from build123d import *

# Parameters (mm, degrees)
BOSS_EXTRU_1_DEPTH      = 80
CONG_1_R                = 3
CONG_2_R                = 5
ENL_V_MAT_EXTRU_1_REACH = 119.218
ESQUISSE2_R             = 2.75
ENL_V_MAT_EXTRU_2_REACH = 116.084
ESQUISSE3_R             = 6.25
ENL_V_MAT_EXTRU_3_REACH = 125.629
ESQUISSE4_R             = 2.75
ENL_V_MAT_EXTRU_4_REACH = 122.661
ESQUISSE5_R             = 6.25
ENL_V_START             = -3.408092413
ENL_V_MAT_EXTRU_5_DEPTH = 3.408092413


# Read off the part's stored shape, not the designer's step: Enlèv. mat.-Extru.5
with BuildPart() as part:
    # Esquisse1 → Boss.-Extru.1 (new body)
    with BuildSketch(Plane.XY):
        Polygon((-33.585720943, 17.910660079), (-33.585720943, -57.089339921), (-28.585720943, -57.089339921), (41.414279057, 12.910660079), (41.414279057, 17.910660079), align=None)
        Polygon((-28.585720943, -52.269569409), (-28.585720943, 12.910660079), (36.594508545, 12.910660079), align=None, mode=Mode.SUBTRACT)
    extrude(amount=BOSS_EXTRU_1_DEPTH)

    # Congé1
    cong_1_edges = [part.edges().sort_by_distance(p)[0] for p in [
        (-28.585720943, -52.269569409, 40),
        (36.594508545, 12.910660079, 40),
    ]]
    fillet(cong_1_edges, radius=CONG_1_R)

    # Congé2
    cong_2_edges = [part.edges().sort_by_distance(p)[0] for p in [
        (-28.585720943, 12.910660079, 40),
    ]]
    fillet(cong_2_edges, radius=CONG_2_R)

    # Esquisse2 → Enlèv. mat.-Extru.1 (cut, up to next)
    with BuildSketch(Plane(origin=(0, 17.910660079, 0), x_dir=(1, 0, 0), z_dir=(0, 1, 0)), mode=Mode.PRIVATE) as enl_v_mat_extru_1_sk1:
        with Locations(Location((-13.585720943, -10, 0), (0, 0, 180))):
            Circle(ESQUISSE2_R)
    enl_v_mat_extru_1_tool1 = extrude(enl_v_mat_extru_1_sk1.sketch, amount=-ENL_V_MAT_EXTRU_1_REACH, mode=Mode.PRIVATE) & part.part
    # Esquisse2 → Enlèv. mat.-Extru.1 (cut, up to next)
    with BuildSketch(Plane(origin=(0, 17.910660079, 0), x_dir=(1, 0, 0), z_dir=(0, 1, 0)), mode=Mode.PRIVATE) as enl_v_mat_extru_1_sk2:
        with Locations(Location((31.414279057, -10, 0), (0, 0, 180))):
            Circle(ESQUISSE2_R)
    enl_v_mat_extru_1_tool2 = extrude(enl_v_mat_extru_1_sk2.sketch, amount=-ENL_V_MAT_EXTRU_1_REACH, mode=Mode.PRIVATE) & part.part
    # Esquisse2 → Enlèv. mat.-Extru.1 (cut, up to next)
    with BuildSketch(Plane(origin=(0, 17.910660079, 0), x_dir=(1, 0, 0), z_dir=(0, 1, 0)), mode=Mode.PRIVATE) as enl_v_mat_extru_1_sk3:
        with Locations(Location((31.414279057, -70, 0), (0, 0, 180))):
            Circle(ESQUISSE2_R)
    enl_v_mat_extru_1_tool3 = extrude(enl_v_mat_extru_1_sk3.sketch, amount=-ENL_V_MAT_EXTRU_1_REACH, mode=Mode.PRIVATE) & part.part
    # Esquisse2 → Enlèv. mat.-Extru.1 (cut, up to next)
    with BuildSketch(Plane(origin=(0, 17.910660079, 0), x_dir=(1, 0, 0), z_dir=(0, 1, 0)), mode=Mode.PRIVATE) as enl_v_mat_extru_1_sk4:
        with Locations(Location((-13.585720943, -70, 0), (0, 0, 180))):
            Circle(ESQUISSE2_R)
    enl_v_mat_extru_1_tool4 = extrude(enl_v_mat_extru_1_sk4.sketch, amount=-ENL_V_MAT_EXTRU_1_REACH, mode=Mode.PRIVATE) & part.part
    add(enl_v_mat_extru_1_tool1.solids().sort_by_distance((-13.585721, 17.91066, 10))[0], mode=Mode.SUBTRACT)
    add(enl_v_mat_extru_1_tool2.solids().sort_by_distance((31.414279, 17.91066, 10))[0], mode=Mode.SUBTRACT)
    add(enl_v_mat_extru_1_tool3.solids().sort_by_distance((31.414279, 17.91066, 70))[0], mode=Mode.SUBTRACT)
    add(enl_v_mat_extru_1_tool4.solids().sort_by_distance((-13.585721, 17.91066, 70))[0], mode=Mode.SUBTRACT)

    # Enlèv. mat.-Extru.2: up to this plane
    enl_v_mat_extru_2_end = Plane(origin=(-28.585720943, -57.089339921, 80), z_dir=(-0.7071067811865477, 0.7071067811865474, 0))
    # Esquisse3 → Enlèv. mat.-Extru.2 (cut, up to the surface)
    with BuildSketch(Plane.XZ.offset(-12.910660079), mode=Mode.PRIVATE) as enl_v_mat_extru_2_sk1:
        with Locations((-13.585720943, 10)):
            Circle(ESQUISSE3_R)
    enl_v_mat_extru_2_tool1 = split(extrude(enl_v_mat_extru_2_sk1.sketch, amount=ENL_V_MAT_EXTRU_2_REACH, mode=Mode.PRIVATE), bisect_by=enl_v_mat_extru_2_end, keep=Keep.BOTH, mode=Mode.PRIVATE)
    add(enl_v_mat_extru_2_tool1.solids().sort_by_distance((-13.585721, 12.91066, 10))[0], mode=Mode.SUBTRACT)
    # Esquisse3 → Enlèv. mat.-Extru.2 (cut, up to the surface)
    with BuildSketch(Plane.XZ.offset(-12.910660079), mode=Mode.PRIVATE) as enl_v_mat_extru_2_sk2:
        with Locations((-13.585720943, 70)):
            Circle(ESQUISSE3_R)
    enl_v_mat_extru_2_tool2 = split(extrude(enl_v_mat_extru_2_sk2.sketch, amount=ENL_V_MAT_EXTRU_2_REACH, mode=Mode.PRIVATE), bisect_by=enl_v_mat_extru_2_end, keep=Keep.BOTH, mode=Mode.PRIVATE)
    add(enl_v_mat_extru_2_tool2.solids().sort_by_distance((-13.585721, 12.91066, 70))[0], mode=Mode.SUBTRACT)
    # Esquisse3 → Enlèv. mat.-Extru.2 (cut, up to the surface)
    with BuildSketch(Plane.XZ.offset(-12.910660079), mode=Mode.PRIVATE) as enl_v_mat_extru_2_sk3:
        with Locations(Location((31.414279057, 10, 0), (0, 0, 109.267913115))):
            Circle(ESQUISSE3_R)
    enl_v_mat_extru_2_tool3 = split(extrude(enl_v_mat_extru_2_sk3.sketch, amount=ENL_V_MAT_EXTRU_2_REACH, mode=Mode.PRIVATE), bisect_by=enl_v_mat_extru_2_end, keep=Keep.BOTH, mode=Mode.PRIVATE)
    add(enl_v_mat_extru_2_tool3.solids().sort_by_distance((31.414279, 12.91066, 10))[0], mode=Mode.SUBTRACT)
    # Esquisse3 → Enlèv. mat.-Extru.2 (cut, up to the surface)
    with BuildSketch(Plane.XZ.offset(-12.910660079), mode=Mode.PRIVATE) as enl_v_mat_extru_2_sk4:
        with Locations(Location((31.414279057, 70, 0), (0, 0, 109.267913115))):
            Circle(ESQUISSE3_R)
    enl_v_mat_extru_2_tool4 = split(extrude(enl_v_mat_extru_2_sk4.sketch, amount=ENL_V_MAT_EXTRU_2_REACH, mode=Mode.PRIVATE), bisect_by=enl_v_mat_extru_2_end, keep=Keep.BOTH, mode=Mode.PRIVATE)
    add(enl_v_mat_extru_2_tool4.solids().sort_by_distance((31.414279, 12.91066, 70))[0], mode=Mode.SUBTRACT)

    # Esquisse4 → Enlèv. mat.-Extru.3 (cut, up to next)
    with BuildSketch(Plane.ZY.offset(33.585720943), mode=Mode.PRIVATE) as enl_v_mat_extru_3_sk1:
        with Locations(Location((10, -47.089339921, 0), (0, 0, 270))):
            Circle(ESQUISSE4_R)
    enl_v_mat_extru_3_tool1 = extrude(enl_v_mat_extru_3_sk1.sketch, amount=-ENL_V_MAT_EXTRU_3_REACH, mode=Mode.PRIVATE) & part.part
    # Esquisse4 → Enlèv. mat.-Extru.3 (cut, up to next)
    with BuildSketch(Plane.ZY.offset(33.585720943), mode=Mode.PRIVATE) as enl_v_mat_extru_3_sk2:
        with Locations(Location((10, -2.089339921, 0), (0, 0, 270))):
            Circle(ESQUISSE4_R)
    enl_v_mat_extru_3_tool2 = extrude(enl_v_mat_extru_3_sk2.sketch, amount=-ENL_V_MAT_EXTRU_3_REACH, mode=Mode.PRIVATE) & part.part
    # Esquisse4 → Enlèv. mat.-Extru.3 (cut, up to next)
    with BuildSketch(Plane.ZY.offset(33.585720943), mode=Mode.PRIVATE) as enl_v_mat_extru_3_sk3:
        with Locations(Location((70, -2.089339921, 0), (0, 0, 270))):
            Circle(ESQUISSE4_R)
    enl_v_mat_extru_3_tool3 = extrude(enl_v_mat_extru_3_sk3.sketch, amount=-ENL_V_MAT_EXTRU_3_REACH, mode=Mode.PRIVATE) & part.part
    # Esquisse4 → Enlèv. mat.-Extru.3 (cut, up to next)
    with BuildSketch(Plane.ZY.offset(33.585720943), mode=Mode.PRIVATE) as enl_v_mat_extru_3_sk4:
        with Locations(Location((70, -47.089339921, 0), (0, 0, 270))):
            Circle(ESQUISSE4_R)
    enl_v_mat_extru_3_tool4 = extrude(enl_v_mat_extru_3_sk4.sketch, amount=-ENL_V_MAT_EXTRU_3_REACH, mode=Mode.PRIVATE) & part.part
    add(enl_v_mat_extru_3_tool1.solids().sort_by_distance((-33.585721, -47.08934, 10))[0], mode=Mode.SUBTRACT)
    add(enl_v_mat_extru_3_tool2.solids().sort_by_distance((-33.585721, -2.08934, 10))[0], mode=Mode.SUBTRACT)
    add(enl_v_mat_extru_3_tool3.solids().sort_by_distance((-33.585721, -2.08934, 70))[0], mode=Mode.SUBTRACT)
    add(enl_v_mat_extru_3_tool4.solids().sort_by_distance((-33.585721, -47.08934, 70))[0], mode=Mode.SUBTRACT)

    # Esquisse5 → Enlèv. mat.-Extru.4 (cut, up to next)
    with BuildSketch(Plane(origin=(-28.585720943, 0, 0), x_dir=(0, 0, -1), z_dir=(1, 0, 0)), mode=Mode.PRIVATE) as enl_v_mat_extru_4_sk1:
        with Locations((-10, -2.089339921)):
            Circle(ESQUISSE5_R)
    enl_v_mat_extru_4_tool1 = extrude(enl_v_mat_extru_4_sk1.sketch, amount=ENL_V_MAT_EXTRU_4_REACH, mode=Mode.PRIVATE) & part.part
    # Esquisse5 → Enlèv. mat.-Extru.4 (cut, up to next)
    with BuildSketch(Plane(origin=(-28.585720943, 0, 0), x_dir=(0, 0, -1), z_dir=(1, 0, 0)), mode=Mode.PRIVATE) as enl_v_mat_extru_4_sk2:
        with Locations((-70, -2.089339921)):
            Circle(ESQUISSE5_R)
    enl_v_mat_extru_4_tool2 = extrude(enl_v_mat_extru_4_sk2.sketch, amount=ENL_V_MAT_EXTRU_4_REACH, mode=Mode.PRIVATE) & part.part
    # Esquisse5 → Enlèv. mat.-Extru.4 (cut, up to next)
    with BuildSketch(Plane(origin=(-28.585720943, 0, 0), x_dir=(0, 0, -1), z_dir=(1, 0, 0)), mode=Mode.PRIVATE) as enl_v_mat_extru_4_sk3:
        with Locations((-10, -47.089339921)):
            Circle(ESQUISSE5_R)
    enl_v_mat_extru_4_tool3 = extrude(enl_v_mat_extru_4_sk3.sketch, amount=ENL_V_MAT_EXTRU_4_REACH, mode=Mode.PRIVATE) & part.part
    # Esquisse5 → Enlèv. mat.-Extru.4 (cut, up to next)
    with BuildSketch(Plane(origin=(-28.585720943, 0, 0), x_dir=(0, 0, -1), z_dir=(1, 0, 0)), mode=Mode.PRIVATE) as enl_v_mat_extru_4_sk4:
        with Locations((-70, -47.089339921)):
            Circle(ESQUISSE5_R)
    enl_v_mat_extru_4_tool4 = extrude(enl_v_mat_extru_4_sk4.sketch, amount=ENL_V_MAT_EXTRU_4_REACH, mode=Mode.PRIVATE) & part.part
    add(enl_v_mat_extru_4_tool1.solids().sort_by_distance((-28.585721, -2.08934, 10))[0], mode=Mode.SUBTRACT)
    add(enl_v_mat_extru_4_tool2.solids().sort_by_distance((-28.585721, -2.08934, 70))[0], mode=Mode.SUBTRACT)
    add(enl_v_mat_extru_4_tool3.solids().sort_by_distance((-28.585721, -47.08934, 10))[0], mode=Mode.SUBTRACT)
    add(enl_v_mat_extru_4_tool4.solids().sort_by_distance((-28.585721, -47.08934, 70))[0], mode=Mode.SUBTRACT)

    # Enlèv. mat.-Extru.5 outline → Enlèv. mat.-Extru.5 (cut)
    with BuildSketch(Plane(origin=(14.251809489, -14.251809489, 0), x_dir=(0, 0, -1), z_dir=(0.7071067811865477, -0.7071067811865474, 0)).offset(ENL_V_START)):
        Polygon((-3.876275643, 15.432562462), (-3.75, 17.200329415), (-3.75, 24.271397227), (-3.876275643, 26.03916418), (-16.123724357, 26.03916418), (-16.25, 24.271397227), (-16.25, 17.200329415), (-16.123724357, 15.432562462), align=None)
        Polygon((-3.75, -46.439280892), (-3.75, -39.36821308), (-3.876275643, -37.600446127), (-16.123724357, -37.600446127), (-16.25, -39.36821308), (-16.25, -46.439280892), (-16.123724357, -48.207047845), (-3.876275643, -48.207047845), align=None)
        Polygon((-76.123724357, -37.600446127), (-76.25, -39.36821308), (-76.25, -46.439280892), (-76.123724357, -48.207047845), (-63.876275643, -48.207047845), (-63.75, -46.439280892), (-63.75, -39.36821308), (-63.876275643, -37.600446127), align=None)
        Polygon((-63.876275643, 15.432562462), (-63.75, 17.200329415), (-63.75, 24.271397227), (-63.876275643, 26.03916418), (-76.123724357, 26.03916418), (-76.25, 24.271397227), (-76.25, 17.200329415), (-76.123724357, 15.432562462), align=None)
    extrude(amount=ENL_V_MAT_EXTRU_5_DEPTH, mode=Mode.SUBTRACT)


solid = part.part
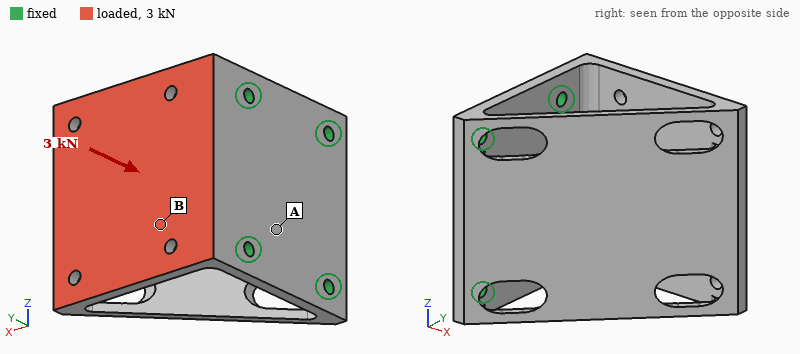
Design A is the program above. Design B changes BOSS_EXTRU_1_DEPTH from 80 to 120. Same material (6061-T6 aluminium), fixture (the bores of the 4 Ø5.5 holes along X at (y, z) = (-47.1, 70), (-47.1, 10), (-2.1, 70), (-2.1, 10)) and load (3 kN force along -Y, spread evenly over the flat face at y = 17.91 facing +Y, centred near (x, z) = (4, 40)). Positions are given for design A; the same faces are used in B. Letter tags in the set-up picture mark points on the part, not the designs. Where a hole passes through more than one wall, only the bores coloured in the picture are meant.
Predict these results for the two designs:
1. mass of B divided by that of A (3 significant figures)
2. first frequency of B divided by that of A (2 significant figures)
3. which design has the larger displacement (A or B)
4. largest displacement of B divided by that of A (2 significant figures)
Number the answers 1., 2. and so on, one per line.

1. 1.53
2. 0.94
3. A
4. 0.72
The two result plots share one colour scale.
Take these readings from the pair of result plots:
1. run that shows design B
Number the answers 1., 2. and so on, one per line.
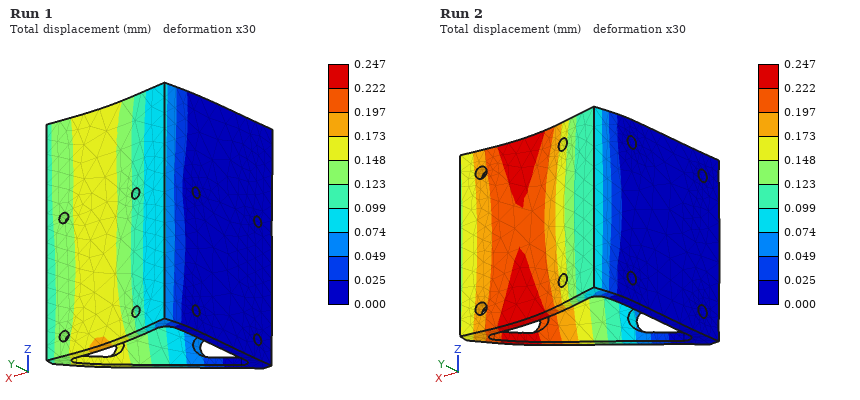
1. Run 1
